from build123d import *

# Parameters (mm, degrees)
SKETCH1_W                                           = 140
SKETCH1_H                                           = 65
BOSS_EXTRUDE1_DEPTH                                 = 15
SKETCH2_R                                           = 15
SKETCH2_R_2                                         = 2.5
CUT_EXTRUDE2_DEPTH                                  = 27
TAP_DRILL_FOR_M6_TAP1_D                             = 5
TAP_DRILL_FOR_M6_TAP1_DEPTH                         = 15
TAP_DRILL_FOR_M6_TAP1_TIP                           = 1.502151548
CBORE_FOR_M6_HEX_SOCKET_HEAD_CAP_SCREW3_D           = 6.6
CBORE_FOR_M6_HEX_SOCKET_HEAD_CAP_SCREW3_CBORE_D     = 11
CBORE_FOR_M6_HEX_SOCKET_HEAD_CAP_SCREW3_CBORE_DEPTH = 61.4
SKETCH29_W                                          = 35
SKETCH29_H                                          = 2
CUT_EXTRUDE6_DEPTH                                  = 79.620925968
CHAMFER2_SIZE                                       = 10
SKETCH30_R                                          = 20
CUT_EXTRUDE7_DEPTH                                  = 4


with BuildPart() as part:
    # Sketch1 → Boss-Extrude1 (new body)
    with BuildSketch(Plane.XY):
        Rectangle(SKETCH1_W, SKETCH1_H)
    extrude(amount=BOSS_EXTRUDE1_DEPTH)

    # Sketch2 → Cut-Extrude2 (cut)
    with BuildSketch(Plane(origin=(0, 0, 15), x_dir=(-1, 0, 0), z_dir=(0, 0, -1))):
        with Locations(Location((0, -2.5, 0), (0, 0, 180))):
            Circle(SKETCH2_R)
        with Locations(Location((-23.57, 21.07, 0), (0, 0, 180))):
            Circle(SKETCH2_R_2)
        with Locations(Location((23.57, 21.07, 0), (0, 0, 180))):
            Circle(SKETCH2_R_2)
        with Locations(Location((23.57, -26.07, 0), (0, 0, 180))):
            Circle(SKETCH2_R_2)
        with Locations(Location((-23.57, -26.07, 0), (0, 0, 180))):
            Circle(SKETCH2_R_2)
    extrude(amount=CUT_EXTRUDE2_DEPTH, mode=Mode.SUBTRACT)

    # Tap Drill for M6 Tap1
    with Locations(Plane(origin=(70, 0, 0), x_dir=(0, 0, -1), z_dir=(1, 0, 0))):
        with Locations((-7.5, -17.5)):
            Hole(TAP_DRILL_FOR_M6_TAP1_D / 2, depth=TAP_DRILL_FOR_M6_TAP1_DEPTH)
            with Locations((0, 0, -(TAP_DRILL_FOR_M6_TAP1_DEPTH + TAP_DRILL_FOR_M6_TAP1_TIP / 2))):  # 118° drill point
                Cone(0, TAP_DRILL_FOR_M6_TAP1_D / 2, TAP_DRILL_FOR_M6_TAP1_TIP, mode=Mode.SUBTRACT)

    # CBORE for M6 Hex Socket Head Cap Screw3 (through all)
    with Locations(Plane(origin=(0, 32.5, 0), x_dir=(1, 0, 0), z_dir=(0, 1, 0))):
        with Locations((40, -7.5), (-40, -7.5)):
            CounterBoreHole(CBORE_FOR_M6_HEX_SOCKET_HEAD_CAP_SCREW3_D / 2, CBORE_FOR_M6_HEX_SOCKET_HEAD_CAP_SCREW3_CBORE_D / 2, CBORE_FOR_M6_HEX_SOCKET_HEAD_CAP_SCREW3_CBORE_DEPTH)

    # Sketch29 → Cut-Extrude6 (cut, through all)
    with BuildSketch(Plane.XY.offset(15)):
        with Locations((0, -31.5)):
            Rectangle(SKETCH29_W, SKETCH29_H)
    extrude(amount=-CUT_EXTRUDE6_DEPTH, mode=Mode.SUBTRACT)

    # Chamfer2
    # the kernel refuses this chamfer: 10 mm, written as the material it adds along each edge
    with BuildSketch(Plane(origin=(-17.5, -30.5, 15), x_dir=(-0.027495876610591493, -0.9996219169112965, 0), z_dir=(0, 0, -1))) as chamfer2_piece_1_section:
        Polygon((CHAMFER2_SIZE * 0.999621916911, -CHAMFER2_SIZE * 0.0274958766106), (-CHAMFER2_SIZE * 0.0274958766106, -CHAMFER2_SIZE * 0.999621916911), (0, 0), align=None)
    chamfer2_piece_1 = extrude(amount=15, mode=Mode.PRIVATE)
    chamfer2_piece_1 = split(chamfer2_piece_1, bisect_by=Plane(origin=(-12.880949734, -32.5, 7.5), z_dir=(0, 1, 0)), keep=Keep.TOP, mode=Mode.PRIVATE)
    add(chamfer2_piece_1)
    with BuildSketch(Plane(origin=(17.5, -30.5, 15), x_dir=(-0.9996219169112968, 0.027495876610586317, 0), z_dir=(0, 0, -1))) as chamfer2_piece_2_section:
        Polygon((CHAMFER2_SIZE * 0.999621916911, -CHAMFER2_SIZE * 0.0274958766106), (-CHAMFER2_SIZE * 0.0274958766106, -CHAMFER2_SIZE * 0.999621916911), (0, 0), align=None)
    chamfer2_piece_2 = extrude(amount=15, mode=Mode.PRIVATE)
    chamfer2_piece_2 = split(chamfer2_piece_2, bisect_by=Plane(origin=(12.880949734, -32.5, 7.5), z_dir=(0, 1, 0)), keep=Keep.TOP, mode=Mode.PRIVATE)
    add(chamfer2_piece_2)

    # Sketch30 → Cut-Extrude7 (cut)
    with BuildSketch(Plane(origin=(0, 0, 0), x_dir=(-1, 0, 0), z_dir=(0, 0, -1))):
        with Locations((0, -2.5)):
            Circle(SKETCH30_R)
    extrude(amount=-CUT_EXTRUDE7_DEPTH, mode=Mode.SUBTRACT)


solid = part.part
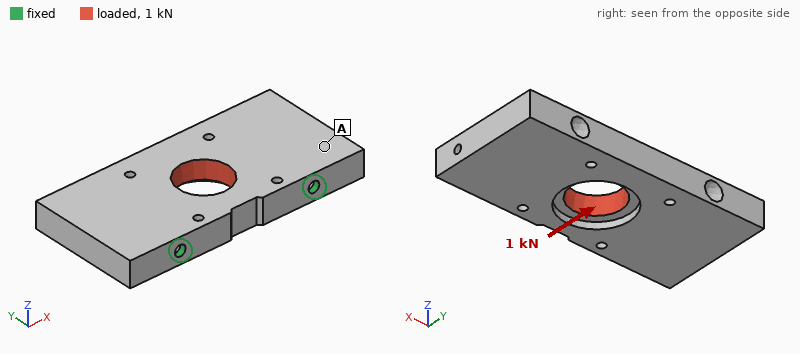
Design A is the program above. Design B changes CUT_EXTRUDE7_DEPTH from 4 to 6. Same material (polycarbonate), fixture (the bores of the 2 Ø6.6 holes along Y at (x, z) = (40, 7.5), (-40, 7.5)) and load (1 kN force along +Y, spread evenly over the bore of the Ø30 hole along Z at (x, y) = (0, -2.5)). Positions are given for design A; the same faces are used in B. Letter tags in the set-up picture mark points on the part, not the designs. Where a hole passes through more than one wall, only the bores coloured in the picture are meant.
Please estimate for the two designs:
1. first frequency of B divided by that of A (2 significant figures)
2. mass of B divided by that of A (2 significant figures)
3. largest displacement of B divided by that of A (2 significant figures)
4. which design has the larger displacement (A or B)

1.0
0.99
1.5
B
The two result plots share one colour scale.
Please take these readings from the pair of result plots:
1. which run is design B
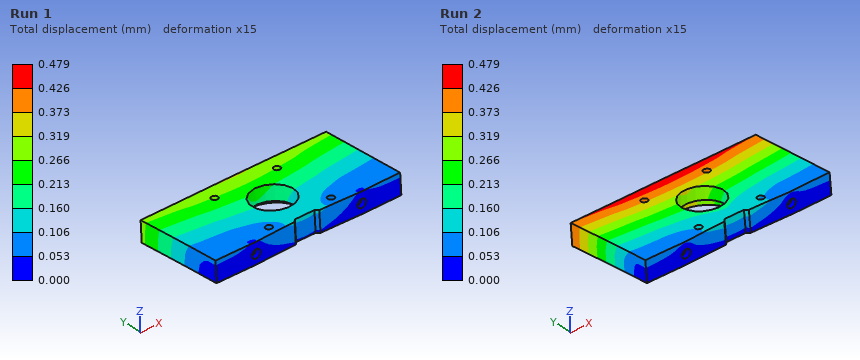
Run 2
